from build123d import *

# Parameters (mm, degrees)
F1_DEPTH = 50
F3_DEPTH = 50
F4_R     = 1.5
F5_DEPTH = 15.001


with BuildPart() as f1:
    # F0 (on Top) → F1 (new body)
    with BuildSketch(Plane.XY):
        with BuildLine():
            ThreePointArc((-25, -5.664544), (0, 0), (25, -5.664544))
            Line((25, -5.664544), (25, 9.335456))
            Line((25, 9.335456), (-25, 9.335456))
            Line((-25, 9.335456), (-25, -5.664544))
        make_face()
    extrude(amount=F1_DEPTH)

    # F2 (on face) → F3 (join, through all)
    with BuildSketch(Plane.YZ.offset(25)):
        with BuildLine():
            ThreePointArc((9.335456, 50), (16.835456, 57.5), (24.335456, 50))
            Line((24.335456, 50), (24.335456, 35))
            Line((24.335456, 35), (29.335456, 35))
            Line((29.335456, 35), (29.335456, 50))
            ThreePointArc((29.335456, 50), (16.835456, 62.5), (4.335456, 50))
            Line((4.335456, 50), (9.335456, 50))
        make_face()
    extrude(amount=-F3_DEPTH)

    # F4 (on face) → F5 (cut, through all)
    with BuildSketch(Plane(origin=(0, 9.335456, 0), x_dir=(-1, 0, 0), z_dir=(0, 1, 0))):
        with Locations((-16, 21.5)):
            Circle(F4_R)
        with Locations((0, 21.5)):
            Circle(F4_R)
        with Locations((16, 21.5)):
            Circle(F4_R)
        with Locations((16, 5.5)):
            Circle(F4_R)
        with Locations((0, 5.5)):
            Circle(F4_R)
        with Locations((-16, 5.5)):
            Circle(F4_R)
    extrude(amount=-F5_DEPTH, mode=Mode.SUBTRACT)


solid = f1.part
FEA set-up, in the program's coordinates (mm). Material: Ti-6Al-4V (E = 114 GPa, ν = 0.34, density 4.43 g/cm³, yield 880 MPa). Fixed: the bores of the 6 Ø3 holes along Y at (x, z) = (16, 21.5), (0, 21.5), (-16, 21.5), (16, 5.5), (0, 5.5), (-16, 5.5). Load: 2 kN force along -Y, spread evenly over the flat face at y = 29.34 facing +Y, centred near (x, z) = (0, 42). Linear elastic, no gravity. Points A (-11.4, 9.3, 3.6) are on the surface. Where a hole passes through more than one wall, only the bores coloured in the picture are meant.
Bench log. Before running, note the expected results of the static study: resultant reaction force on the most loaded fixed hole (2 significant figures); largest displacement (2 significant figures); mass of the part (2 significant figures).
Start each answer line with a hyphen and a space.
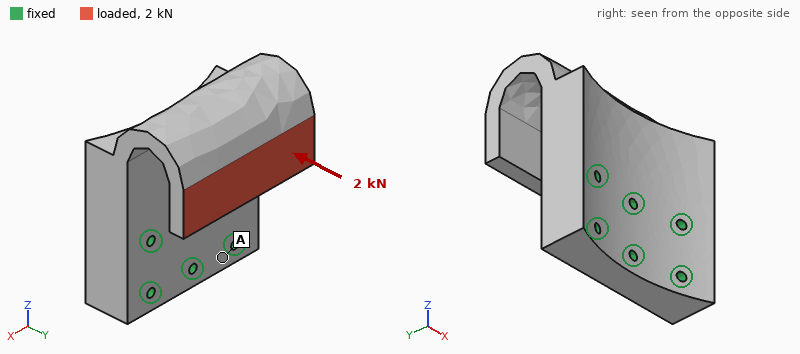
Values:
- 1.1 kN
- 0.35 mm
- 170 g
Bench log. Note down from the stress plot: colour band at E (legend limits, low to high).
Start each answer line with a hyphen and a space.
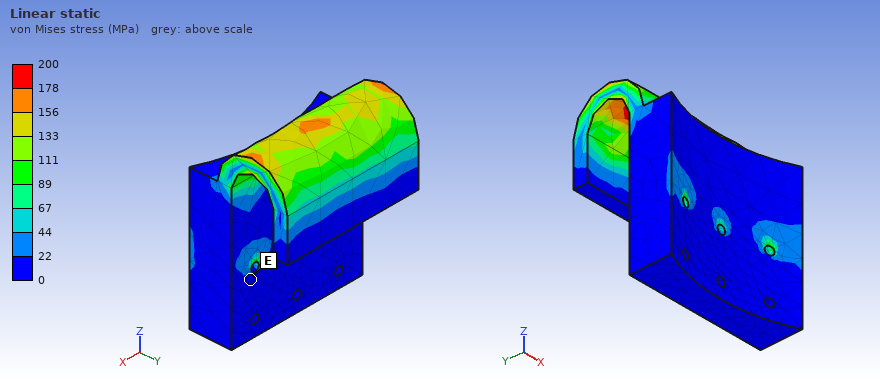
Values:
- 0 to 22 MPa
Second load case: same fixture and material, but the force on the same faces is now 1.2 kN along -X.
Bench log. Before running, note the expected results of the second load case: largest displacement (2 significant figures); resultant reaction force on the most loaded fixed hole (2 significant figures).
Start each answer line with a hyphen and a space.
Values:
- 0.13 mm
- 1.1 kN
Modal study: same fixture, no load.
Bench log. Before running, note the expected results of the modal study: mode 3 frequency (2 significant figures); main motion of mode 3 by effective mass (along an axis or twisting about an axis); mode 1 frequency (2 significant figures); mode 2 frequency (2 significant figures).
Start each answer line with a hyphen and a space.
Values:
- 3700 Hz
- along Y
- 2400 Hz
- 3300 Hz
